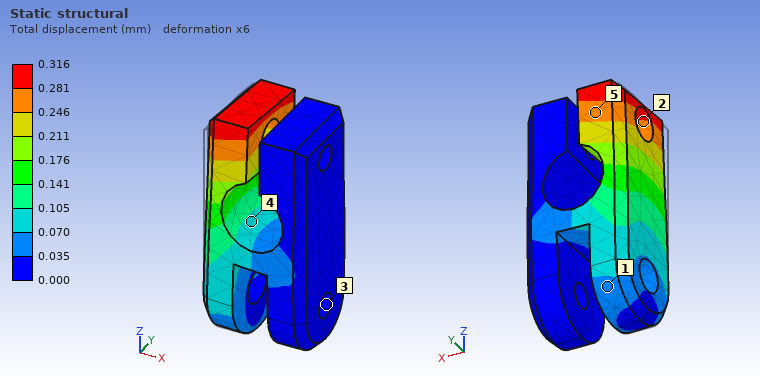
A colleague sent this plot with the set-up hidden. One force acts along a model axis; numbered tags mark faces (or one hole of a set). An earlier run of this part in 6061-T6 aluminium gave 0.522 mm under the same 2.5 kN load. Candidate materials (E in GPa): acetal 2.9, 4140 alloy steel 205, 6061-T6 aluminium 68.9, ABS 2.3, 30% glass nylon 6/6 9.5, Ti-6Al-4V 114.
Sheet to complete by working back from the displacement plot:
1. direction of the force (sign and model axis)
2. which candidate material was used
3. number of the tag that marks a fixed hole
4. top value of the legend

+Y
Ti-6Al-4V
3
0.316 mm
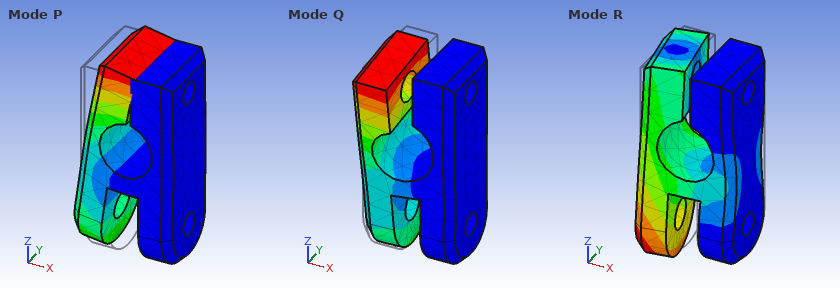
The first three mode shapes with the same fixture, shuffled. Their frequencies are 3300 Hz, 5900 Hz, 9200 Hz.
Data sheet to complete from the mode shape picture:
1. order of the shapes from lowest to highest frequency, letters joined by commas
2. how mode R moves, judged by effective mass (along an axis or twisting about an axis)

P, Q, R
along Y
